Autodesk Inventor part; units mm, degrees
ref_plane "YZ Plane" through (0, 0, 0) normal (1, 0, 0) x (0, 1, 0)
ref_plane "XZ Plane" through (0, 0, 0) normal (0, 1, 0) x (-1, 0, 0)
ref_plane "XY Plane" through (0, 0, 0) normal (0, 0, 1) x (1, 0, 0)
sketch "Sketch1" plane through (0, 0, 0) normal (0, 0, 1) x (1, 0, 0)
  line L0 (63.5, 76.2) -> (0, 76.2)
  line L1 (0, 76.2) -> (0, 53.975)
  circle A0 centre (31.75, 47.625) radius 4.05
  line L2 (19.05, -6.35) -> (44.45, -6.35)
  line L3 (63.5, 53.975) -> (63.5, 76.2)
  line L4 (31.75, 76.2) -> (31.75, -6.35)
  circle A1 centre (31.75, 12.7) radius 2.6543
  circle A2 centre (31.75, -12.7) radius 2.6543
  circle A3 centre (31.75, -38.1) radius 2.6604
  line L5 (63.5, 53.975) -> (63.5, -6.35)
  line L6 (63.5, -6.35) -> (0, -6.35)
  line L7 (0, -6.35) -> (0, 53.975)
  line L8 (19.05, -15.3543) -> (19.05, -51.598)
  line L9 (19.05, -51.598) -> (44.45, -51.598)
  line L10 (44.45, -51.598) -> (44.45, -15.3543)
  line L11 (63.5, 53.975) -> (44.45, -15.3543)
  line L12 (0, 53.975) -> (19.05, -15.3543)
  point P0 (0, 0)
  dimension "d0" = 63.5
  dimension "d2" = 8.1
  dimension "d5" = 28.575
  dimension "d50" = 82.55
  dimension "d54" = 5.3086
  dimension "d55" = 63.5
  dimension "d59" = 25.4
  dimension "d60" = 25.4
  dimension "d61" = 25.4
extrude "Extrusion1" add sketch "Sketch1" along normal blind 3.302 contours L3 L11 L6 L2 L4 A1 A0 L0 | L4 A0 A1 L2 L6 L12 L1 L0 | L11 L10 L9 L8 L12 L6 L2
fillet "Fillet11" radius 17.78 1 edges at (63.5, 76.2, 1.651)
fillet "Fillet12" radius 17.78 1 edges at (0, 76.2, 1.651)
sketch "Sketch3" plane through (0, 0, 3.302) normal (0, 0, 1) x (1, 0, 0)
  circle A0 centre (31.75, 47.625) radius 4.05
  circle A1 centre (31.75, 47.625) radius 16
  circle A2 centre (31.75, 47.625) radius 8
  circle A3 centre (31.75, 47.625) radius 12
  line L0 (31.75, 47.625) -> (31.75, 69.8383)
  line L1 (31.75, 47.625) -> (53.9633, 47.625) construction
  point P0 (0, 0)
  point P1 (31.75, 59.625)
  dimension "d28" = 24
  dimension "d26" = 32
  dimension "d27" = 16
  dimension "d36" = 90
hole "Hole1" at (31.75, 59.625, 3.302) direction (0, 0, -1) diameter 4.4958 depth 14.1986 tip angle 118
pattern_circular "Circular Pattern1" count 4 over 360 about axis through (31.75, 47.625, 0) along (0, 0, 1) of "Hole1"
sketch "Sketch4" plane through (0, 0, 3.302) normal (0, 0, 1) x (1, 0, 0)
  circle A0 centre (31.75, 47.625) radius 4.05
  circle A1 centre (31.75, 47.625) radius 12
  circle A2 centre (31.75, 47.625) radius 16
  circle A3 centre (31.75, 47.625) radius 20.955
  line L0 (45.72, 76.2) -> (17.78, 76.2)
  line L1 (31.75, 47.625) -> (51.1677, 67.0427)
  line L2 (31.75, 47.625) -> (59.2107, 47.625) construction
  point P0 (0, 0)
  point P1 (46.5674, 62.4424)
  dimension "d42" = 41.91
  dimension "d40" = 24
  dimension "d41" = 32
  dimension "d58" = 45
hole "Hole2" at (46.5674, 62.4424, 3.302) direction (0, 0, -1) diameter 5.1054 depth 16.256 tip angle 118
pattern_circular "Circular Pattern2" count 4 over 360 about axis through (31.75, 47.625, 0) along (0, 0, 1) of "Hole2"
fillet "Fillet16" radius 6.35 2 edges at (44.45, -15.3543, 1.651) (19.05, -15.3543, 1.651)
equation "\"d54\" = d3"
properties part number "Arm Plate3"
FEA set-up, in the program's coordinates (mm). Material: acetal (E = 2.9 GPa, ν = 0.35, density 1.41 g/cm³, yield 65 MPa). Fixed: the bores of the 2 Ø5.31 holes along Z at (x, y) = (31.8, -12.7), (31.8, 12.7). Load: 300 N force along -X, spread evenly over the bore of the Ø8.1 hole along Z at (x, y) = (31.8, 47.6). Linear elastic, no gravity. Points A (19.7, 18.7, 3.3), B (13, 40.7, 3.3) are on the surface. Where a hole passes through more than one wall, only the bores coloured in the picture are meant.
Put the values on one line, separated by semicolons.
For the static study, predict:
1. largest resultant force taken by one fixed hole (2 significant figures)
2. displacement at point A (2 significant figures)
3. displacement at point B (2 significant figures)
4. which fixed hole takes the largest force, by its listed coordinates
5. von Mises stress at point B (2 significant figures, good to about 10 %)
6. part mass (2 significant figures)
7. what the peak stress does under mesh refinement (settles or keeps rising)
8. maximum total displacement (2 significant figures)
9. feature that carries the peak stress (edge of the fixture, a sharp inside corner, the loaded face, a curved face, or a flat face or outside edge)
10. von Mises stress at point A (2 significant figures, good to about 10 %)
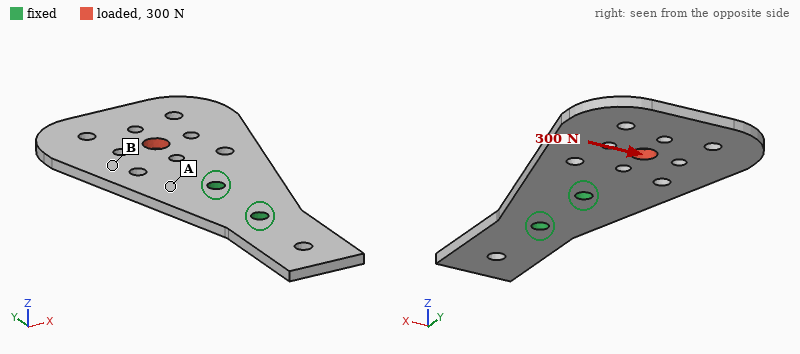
630 N; 0.097 mm; 0.32 mm; (31.8, 12.7); 2.8 MPa; 23 g; keeps rising; 0.62 mm; edge of the fixture; 6.4 MPa
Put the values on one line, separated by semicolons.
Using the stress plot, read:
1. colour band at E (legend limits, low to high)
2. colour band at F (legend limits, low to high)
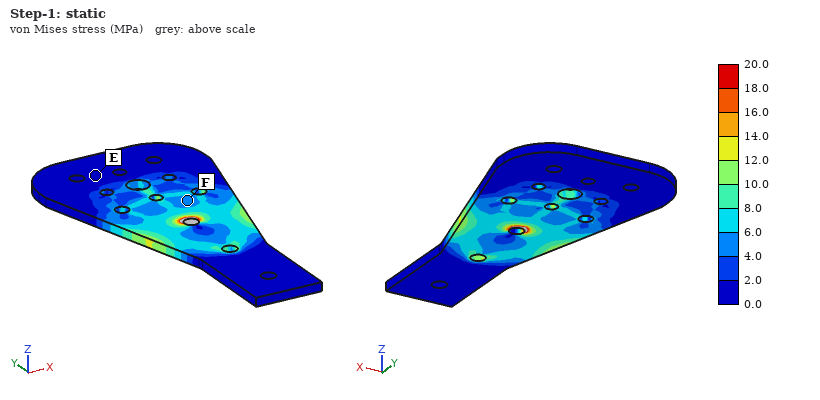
0.0 to 2.0 MPa; 4.0 to 6.0 MPa
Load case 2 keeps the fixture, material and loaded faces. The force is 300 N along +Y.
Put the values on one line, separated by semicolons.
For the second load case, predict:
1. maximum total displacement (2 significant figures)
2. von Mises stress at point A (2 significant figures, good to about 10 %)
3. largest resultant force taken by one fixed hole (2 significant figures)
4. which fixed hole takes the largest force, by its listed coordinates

53 µm; 1.6 MPa; 220 N; (31.8, 12.7)
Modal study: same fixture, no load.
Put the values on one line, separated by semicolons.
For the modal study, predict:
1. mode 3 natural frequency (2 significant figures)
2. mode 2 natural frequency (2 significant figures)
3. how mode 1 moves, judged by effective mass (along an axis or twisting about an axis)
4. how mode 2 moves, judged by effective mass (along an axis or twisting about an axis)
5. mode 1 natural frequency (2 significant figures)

540 Hz; 350 Hz; along Z; twisting about Y; 170 Hz
